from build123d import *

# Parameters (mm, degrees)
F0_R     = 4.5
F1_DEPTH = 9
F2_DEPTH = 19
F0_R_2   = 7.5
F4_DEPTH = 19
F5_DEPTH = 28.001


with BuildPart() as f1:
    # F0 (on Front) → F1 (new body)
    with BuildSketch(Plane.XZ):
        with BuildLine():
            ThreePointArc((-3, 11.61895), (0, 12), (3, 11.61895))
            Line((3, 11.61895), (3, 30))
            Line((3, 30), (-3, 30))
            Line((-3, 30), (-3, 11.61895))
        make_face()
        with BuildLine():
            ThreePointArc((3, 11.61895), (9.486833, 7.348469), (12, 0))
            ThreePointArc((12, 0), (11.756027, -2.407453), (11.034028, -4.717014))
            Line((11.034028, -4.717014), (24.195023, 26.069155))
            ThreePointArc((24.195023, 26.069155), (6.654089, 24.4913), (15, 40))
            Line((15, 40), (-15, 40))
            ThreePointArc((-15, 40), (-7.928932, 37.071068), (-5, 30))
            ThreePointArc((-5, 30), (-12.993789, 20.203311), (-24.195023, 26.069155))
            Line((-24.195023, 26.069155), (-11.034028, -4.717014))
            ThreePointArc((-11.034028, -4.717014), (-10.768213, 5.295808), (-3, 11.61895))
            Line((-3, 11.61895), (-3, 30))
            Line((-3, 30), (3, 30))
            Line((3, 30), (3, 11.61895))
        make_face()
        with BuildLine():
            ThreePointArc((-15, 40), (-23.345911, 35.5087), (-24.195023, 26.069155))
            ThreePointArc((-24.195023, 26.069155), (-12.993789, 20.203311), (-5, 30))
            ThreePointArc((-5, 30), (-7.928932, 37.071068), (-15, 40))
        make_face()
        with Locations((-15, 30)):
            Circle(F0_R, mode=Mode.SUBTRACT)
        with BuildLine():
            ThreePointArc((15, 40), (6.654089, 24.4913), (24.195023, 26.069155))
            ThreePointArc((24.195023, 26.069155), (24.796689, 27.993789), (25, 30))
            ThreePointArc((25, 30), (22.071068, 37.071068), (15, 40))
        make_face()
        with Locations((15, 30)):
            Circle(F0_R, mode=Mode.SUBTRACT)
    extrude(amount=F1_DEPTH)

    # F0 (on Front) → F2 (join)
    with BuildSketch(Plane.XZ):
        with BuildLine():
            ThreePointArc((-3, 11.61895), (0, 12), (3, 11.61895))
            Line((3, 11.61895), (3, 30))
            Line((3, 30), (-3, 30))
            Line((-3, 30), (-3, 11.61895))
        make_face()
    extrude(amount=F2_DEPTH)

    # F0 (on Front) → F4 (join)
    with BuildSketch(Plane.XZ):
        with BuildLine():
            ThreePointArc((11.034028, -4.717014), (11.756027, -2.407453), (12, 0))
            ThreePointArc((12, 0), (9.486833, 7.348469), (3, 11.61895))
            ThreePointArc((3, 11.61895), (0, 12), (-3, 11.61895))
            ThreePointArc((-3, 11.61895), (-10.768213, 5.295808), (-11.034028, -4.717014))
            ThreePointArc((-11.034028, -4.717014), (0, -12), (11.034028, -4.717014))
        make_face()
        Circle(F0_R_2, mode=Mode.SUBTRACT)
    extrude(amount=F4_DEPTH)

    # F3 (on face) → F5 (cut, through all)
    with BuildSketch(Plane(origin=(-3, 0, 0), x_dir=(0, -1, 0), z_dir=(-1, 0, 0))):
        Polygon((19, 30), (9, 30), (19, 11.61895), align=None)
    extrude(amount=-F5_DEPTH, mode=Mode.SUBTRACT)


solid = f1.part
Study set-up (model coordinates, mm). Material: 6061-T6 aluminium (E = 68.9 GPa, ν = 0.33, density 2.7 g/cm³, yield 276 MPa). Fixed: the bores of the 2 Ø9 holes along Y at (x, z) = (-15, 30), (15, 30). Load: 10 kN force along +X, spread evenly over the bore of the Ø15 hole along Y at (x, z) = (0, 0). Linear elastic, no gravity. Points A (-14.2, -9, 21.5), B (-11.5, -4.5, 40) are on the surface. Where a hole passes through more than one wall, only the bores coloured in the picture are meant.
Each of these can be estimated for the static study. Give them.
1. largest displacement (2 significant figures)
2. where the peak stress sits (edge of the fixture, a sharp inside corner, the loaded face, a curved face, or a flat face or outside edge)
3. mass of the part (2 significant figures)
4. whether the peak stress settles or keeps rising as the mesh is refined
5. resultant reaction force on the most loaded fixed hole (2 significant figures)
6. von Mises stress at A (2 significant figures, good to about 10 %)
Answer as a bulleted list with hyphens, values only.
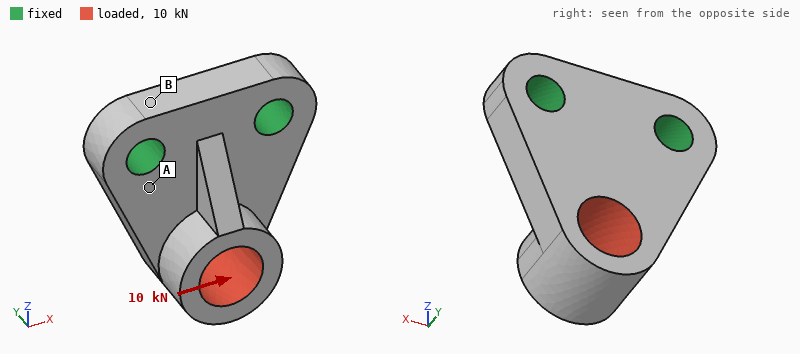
- 0.13 mm
- edge of the fixture
- 47 g
- keeps rising
- 9.9 kN
- 58 MPa
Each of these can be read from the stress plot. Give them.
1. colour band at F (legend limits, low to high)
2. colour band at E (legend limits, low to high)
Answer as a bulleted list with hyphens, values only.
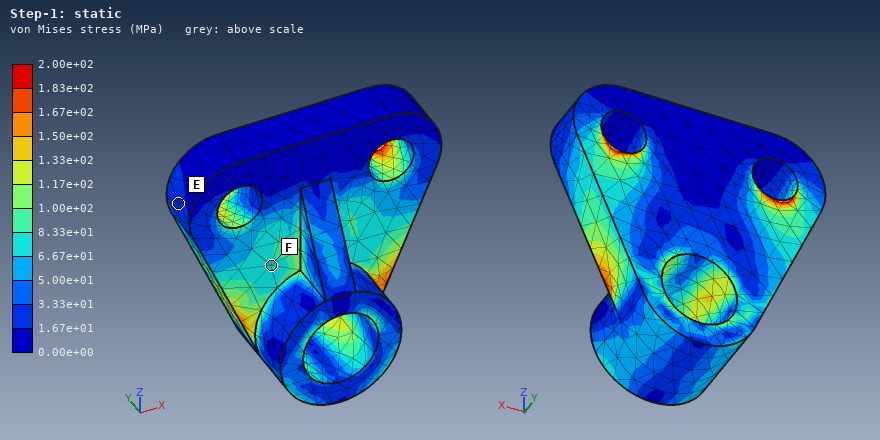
- 6.67e+01 to 8.33e+01 MPa
- 1.67e+01 to 3.33e+01 MPa
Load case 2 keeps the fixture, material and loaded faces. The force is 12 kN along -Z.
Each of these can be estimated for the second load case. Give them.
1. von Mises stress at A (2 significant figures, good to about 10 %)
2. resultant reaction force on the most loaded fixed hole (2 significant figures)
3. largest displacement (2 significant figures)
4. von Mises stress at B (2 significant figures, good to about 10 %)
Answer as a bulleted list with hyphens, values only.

- 130 MPa
- 6.2 kN
- 0.23 mm
- 22 MPa
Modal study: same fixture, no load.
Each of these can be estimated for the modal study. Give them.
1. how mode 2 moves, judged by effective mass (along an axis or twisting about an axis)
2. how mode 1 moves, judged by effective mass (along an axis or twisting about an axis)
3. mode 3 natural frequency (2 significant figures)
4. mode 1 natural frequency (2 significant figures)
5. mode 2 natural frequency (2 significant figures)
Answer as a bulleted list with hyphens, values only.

- along X
- along Y
- 16 kHz
- 5500 Hz
- 13 kHz
